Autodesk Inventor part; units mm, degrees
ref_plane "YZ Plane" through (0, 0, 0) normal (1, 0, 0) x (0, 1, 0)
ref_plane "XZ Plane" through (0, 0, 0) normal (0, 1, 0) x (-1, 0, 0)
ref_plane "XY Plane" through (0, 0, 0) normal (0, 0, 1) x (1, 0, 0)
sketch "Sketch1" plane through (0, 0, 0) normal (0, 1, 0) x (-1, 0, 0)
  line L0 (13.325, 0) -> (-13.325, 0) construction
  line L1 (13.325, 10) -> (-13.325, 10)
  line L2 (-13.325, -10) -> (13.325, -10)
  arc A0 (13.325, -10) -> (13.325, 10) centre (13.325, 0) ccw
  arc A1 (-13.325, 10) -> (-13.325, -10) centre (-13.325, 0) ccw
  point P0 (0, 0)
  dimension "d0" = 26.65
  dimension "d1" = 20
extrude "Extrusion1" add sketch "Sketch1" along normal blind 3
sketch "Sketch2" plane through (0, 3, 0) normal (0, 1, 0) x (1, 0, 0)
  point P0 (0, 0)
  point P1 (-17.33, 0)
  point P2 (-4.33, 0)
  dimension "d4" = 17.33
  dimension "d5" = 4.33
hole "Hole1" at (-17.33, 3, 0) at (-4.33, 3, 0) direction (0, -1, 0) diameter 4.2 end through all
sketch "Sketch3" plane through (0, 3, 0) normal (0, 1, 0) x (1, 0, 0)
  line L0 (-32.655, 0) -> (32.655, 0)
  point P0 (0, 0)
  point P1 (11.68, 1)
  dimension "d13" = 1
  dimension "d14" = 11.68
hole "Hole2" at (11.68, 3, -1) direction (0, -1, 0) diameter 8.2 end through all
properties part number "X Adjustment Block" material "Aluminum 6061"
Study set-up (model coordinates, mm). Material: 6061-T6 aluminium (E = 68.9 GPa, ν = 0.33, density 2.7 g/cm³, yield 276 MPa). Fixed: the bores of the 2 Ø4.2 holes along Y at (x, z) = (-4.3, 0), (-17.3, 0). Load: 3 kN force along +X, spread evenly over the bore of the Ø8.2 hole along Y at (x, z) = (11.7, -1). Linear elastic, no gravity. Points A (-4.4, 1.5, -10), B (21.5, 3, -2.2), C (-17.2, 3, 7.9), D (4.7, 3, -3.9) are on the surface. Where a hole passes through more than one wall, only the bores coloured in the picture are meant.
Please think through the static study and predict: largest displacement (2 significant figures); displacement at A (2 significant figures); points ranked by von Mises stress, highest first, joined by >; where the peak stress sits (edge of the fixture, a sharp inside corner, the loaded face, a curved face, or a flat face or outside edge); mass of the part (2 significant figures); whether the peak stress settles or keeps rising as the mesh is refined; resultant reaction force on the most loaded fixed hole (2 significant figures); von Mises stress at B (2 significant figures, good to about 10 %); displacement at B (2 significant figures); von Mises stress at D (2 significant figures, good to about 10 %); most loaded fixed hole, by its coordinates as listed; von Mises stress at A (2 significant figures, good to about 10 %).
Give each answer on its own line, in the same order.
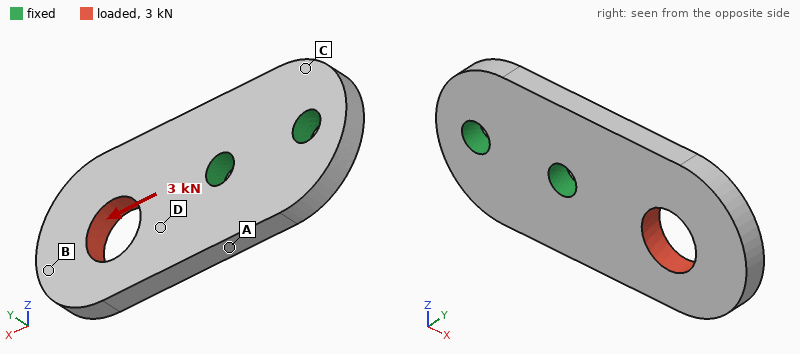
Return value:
28 µm
7.7 µm
D > A > B > C
edge of the fixture
6.2 g
keeps rising
2.4 kN
33 MPa
26 µm
67 MPa
(-4.3, 0)
47 MPa
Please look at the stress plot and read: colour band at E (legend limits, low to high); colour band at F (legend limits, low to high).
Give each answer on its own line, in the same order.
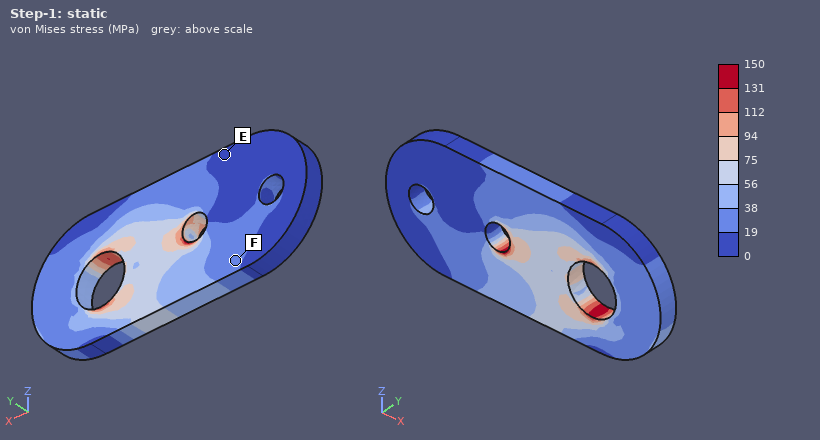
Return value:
0 to 19 MPa
19 to 38 MPa
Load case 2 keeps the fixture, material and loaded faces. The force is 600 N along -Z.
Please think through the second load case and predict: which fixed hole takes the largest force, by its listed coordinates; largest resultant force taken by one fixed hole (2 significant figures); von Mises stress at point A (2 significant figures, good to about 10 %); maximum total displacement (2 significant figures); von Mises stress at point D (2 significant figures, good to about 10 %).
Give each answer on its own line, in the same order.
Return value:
(-4.3, 0)
1.1 kN
44 MPa
41 µm
23 MPa
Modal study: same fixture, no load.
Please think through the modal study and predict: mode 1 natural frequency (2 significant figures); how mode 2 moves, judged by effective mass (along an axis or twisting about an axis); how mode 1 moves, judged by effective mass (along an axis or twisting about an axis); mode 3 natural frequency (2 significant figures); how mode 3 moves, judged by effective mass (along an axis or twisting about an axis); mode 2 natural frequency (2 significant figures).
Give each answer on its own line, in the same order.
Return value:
3900 Hz
twisting about X
along Y
13 kHz
along Z
9400 Hz
